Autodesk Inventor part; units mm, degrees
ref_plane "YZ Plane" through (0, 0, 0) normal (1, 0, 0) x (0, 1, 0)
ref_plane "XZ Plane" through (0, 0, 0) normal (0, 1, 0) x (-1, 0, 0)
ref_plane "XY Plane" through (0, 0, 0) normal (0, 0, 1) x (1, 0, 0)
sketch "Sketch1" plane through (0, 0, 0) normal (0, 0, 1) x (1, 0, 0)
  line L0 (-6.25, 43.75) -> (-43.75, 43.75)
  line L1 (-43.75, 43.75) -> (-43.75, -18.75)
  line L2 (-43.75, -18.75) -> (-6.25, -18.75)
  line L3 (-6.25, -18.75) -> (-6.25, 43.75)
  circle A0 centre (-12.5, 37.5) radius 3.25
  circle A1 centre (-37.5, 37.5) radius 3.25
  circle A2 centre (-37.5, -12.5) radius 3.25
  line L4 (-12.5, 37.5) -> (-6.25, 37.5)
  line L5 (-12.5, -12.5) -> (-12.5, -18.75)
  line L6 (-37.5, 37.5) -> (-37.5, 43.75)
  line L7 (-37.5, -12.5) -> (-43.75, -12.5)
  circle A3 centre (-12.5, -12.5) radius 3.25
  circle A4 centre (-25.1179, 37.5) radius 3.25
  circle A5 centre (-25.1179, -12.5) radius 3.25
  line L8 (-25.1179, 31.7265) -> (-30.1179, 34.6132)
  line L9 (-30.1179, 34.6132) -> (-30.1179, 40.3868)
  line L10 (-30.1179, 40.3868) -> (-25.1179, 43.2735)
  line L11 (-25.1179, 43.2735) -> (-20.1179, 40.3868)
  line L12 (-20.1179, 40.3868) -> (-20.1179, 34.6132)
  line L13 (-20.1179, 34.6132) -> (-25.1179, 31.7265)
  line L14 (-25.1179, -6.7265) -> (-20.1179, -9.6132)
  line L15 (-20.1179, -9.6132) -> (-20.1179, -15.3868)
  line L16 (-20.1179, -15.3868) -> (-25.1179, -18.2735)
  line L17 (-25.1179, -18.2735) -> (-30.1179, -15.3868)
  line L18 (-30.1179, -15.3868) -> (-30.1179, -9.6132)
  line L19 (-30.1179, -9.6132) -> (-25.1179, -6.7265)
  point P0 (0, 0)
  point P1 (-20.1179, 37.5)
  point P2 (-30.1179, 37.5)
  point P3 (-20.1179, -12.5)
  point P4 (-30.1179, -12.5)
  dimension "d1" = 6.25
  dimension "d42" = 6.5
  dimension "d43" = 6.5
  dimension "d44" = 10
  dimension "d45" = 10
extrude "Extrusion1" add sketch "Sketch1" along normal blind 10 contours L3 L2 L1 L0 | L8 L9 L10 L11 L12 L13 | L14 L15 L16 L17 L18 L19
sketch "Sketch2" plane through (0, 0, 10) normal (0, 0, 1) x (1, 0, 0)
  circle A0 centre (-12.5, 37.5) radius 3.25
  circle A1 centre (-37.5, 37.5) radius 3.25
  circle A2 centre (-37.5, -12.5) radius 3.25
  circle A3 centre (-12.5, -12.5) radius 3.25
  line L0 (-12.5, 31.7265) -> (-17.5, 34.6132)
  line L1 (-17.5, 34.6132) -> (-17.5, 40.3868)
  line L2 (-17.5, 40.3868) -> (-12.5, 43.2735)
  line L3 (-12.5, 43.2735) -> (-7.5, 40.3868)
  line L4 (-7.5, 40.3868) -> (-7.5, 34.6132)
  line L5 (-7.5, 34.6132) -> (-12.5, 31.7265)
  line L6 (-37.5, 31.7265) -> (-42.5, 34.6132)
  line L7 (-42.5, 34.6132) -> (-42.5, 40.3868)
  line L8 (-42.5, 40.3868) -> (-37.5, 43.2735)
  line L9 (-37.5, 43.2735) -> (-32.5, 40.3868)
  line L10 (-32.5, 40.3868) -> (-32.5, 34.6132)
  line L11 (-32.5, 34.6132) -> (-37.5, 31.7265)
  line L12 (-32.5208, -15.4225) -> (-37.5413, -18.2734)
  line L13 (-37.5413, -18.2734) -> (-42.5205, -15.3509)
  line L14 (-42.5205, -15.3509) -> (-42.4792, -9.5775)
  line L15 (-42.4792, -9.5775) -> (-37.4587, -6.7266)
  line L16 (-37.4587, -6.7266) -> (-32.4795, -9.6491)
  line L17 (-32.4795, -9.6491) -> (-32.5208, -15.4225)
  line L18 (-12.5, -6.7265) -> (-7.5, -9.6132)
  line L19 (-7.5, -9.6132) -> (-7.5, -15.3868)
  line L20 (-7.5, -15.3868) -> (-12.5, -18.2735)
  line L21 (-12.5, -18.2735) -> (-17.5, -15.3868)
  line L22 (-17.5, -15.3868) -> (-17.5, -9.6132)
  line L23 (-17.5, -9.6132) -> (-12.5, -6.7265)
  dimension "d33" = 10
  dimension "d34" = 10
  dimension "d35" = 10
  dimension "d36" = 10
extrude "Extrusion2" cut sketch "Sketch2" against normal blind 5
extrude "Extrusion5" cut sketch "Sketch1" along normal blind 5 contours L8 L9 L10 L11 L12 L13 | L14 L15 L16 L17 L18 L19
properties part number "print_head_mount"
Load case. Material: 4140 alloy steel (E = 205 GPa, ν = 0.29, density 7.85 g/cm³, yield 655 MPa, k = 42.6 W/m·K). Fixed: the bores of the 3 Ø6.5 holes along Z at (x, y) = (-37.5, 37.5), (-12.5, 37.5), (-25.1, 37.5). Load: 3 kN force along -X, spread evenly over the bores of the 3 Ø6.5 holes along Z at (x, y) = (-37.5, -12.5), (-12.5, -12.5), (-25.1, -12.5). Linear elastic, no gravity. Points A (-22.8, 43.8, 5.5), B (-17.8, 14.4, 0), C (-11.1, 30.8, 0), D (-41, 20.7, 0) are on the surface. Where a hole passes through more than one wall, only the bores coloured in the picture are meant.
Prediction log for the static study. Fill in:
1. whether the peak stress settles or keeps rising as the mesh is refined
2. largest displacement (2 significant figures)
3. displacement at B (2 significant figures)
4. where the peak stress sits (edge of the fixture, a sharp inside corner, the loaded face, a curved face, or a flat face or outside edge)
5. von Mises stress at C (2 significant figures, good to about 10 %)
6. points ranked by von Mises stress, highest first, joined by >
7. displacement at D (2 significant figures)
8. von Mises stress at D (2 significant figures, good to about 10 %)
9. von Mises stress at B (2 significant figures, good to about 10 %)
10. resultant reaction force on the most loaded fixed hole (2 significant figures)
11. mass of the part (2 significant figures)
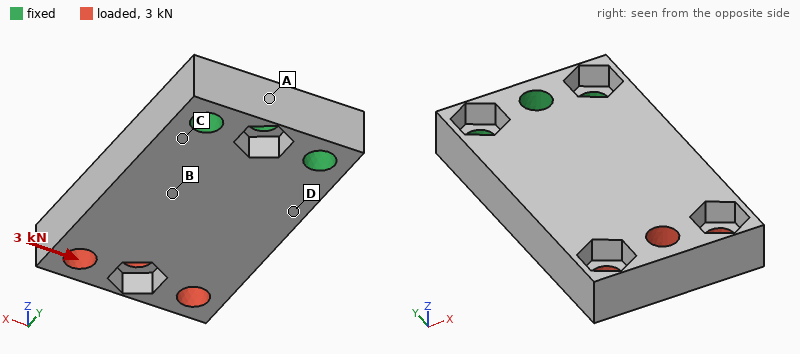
keeps rising
34 µm
10 µm
edge of the fixture
67 MPa
C > D > B > A
8.7 µm
49 MPa
32 MPa
5.2 kN
160 g
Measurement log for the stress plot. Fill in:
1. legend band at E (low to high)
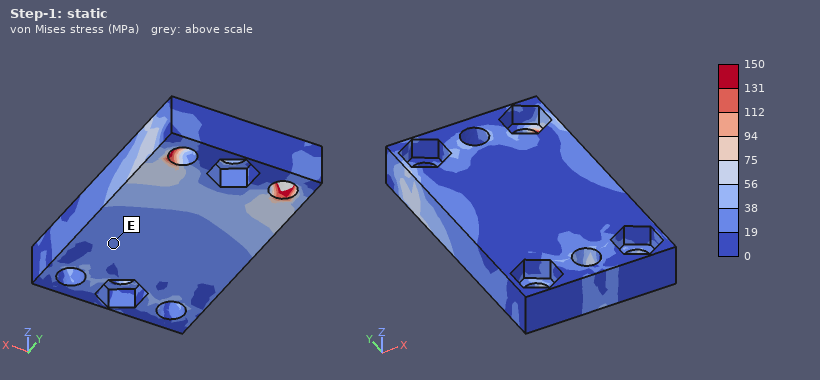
19 to 38 MPa
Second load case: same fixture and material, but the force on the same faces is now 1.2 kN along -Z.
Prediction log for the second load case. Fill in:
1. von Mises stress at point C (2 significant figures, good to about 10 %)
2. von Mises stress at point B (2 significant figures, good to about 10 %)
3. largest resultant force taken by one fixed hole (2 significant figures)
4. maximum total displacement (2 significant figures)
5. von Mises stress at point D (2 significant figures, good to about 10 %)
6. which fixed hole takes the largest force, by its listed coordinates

120 MPa
48 MPa
5.5 kN
0.11 mm
69 MPa
(-25.1, 37.5)
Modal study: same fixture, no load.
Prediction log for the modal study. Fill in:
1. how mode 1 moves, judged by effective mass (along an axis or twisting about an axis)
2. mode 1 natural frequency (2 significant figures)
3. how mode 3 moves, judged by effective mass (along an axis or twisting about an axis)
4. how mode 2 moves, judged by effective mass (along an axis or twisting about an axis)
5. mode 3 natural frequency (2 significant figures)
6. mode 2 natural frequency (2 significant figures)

along Z
2600 Hz
along X
along X
8400 Hz
7100 Hz
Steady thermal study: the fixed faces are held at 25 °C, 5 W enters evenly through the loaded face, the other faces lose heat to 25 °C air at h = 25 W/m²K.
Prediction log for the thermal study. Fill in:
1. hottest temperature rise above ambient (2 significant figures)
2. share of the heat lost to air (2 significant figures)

16 K
25 %
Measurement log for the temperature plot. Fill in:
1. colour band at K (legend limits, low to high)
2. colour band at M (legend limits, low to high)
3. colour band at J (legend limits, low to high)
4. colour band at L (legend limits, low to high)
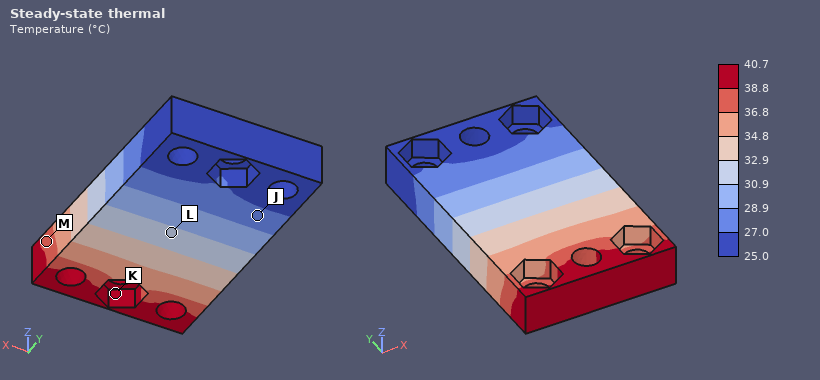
38.8 to 40.7 °C
36.8 to 38.8 °C
27.0 to 28.9 °C
30.9 to 32.9 °C
